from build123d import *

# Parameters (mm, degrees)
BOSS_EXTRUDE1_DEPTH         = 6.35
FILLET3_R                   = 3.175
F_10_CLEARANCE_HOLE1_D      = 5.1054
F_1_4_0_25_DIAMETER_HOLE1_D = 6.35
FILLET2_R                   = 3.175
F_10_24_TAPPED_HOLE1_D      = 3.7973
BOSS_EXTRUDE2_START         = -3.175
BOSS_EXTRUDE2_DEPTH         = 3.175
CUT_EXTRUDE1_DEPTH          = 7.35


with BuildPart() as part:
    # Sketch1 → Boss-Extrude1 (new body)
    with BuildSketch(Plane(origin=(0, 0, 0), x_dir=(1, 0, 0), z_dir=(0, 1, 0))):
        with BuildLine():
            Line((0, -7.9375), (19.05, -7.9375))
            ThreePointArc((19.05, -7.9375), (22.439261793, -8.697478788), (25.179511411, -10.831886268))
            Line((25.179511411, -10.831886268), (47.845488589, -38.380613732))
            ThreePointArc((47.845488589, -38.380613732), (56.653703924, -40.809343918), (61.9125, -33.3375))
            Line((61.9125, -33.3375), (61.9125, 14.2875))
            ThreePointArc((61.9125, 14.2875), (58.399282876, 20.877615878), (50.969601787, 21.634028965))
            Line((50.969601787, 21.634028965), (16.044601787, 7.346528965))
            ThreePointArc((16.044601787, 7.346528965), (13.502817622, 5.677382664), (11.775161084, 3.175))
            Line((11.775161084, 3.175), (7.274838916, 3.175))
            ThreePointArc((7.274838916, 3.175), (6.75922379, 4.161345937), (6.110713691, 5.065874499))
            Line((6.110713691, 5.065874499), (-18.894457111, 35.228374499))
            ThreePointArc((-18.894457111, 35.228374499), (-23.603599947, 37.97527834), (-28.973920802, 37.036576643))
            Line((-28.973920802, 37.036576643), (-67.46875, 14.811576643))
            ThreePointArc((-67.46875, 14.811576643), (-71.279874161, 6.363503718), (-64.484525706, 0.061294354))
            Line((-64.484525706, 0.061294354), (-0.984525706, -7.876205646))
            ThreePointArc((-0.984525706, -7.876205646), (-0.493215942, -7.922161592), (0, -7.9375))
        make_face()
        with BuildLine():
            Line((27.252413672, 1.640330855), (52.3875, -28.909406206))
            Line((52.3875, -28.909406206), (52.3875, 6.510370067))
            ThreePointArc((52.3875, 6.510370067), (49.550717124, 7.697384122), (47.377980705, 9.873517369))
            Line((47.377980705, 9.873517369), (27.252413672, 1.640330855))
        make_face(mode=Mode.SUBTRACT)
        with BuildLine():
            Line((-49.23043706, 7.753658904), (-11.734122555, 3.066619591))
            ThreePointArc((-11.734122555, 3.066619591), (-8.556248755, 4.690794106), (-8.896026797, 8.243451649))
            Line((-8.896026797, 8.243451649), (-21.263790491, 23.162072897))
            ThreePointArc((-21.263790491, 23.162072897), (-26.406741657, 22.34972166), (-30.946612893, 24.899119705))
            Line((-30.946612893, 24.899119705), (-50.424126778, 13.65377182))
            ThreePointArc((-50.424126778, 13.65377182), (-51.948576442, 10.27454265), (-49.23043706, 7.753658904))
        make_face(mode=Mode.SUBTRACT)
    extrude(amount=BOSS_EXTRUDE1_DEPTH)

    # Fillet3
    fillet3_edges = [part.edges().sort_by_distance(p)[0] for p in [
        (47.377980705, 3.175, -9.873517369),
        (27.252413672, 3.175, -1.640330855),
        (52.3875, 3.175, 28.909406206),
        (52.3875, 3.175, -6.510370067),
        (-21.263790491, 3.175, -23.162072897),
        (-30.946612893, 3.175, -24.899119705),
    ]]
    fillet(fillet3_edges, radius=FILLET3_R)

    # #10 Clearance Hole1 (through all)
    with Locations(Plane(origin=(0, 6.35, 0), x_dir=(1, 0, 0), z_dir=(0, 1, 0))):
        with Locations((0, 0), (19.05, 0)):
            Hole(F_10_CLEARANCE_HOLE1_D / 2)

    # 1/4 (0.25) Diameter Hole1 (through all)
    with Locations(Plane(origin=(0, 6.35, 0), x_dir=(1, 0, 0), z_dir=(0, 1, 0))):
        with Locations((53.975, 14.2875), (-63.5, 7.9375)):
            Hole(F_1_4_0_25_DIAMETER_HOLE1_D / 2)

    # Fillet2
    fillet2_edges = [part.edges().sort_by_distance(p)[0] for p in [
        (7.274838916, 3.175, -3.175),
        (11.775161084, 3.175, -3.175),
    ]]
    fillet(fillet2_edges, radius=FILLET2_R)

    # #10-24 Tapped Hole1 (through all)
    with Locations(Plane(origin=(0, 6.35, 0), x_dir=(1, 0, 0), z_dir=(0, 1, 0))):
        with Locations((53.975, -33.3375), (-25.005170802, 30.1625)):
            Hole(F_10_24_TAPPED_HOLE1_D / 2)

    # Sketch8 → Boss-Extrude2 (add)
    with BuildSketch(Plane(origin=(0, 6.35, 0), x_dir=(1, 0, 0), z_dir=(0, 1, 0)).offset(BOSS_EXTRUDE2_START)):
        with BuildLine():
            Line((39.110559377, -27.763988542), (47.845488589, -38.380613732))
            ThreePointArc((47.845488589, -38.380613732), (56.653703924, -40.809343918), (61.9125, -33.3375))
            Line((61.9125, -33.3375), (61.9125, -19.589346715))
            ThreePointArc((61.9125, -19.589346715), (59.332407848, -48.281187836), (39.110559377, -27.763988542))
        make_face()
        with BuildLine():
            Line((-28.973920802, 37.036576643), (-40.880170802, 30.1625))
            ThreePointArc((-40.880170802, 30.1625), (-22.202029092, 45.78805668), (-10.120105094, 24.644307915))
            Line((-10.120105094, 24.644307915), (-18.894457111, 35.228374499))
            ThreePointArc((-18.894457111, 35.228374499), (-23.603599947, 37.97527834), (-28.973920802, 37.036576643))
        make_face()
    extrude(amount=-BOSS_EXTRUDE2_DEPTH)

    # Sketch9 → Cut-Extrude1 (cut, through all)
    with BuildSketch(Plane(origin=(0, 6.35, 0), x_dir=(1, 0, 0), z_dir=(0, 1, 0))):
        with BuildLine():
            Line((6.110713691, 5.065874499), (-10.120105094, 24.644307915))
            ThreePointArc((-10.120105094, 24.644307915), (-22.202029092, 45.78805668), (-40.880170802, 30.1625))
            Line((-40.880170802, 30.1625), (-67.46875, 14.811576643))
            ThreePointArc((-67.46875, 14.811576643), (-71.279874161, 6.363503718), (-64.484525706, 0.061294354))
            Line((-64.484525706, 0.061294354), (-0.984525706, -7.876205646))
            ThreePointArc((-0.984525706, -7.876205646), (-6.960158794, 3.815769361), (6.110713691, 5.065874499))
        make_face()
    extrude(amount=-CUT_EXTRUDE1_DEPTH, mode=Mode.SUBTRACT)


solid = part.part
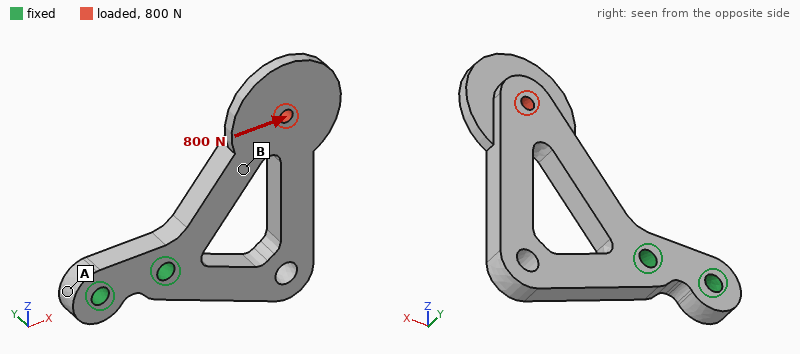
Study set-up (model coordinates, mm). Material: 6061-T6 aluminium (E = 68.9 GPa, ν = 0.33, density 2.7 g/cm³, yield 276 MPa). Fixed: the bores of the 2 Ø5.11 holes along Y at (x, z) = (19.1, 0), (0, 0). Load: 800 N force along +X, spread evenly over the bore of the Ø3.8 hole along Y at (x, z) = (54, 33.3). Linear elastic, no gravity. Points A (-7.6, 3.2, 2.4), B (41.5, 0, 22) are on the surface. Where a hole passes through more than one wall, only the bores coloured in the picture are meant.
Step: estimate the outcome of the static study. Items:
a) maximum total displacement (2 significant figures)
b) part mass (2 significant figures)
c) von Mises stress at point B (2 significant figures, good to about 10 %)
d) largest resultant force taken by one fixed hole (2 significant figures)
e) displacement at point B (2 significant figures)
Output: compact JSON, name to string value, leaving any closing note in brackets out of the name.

{"maximum total displacement": "0.30 mm", "part mass": "32 g", "von Mises stress at point B": "29 MPa", "largest resultant force taken by one fixed hole": "770 N", "displacement at point B": "0.13 mm"}
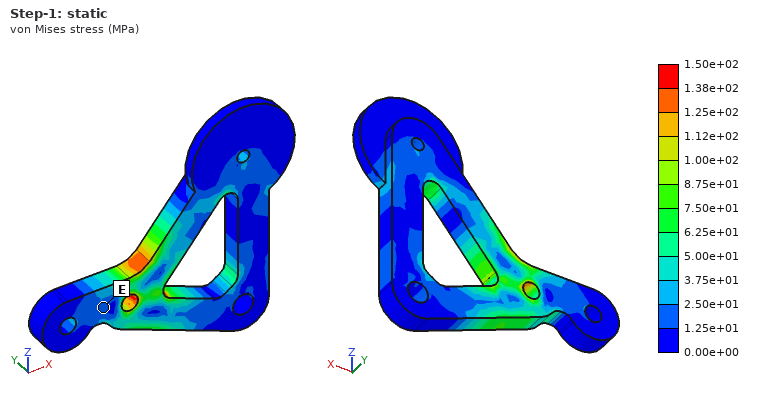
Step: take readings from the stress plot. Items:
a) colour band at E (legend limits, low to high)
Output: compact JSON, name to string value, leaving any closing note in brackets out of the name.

{"colour band at E": "1.25e+01 to 2.50e+01 MPa"}
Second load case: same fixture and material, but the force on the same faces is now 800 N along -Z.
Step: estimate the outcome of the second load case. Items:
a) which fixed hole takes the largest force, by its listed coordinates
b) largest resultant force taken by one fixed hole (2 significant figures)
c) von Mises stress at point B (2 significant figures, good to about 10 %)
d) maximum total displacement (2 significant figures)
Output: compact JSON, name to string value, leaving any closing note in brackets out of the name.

{"which fixed hole takes the largest force, by its listed coordinates": "(19.1, 0)", "largest resultant force taken by one fixed hole": "1.5 kN", "von Mises stress at point B": "19 MPa", "maximum total displacement": "0.29 mm"}
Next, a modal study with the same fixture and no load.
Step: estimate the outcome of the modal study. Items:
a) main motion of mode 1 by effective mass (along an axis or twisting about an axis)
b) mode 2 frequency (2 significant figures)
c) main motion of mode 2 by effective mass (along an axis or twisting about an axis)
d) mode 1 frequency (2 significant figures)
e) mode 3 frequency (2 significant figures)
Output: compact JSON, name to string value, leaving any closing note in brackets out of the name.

{"main motion of mode 1 by effective mass": "along Y", "mode 2 frequency": "2100 Hz", "main motion of mode 2 by effective mass": "along Z", "mode 1 frequency": "1200 Hz", "mode 3 frequency": "2300 Hz"}
